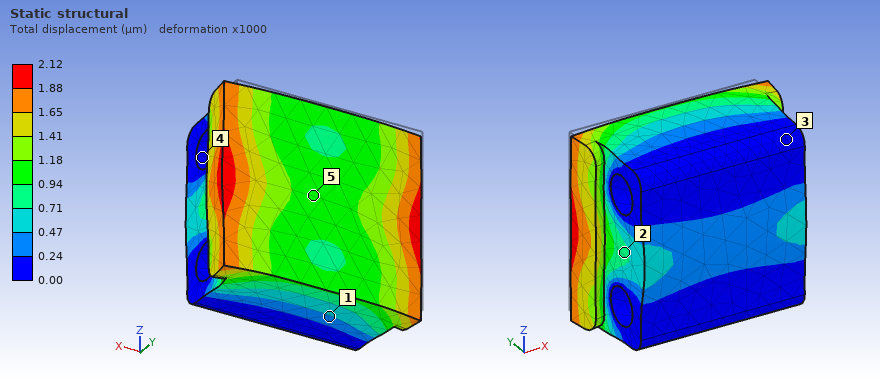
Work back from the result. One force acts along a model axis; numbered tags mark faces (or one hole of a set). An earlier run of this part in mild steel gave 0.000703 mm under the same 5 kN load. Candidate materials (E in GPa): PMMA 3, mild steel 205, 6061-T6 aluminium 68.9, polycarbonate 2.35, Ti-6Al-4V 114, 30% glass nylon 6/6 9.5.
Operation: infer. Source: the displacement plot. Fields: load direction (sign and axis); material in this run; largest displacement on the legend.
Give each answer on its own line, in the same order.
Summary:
-Y
6061-T6 aluminium
2.12 µm
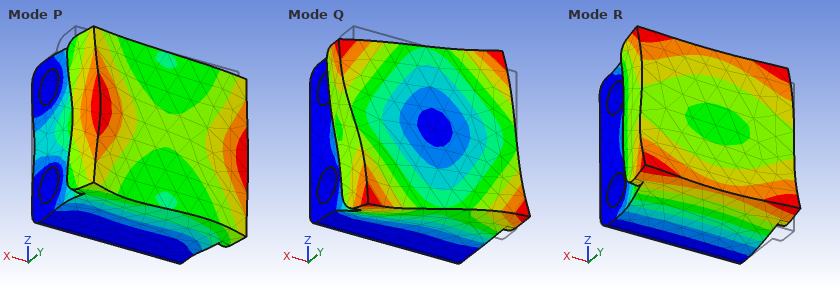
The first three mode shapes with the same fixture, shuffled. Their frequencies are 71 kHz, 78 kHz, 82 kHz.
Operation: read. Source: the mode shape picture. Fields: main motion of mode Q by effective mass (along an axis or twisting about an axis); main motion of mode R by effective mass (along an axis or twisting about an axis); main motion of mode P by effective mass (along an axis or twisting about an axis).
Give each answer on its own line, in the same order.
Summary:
twisting about Y
along Z
along X
